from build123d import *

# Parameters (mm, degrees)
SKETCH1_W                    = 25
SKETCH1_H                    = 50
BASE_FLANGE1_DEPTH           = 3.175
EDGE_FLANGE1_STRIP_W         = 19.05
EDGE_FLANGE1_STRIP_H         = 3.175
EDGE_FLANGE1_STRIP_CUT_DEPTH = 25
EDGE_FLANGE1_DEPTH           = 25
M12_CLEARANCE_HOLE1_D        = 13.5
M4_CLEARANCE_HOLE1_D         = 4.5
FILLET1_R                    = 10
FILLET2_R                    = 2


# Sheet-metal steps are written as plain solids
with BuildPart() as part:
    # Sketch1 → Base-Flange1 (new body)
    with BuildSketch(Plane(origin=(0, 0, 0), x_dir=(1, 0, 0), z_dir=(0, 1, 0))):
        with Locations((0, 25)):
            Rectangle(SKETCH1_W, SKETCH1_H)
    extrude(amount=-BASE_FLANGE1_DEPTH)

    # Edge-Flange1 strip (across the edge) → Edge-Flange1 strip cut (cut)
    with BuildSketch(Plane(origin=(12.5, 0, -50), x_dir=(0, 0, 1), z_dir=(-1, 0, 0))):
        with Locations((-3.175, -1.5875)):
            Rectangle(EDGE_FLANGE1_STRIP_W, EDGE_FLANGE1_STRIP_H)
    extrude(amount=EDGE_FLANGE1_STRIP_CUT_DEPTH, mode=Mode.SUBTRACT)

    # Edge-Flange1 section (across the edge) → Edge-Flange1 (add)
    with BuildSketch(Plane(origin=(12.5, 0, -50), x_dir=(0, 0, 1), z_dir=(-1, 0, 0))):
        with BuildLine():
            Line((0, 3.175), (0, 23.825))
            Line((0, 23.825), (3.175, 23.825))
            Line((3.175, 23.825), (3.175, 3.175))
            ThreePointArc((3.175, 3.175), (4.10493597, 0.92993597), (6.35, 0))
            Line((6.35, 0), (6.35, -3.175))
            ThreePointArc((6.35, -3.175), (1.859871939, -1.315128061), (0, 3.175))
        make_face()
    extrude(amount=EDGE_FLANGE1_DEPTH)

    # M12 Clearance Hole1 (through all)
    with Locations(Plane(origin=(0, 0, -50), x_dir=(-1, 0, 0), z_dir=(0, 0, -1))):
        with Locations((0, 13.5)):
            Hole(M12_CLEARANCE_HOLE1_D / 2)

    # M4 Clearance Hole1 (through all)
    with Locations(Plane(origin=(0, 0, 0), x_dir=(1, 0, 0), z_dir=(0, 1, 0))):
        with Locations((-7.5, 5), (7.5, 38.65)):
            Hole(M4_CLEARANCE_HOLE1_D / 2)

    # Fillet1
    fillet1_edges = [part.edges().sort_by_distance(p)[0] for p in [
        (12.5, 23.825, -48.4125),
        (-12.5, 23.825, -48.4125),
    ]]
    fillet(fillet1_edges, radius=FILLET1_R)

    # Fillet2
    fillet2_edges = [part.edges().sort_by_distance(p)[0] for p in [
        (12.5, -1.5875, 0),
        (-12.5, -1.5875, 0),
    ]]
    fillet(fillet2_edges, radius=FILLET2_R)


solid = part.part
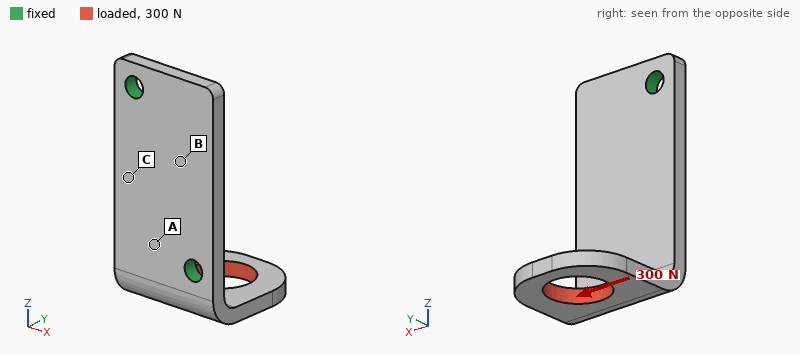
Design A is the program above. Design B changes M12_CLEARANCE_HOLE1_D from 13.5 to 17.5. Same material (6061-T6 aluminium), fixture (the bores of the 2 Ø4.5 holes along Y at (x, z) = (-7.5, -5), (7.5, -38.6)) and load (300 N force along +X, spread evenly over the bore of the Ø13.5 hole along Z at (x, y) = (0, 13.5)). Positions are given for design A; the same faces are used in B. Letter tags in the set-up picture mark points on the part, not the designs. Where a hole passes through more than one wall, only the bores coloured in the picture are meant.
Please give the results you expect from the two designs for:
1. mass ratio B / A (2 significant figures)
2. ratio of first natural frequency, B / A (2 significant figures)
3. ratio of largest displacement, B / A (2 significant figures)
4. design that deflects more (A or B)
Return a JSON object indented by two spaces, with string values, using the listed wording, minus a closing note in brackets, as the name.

{
  "mass ratio B / A": "0.94",
  "ratio of first natural frequency, B / A": "1.1",
  "ratio of largest displacement, B / A": "1.1",
  "design that deflects more": "B"
}
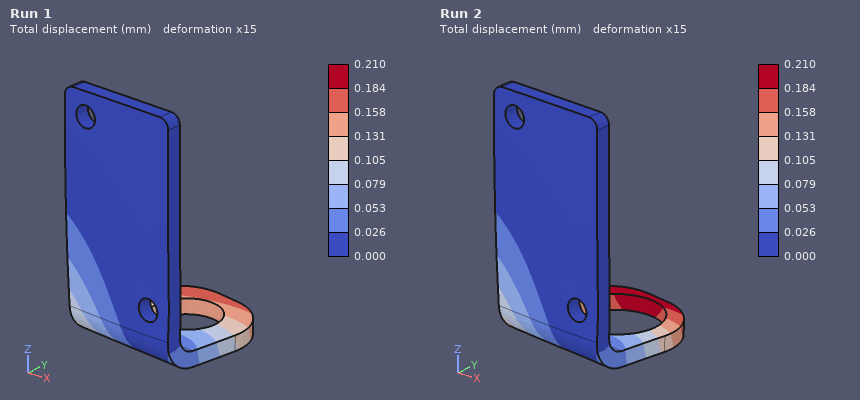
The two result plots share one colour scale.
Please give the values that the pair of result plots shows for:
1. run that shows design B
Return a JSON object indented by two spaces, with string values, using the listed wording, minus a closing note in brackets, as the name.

{
  "run that shows design B": "Run 2"
}
